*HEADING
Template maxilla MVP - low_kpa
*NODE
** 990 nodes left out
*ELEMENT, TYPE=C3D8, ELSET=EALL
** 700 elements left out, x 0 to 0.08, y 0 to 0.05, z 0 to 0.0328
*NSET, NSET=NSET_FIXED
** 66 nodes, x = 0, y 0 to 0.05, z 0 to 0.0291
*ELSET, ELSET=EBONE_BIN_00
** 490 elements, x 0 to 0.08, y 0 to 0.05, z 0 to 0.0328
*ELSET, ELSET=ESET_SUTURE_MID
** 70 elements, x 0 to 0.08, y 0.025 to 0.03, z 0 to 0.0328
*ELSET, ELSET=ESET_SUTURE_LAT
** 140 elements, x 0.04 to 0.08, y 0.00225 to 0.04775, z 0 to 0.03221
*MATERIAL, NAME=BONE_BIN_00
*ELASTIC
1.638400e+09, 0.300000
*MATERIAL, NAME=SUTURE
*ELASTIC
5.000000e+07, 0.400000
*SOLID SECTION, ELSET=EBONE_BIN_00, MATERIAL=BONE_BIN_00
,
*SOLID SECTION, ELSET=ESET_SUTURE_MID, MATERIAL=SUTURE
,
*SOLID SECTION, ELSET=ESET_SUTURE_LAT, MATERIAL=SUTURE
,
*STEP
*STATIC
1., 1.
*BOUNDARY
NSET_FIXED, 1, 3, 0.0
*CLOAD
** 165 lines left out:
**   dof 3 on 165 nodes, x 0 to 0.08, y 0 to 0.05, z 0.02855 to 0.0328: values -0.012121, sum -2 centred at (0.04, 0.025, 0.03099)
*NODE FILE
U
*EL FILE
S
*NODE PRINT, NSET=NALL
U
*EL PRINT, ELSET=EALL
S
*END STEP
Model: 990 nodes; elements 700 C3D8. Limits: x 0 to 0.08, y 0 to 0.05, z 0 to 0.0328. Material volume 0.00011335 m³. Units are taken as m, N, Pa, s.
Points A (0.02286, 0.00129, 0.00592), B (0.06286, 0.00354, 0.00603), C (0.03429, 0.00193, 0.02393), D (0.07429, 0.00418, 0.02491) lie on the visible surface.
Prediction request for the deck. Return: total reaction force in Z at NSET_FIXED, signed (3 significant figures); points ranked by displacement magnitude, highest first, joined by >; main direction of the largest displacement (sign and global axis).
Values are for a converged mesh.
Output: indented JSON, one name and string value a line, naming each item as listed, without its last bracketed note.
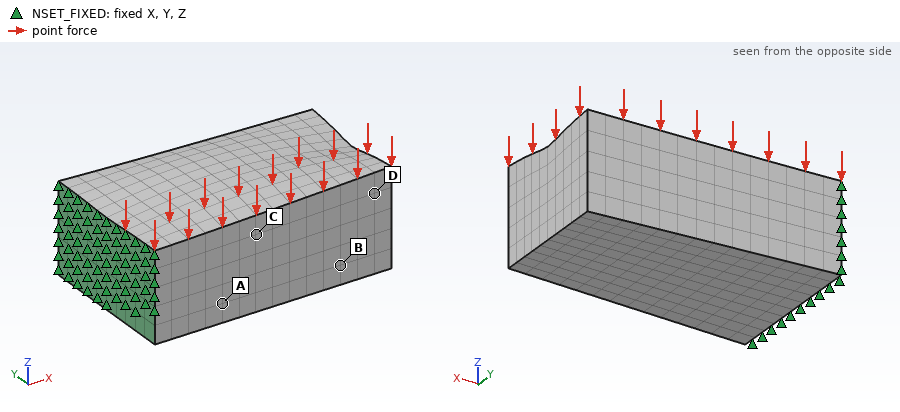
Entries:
{
  "total reaction force in Z at NSET_FIXED, signed": "2.00 N",
  "points ranked by displacement magnitude, highest first, joined by >": "D > B > C > A",
  "main direction of the largest displacement": "-Z"
}
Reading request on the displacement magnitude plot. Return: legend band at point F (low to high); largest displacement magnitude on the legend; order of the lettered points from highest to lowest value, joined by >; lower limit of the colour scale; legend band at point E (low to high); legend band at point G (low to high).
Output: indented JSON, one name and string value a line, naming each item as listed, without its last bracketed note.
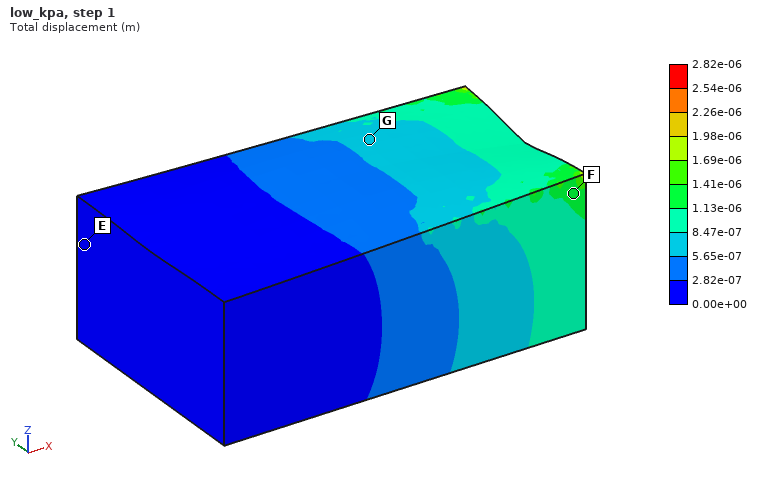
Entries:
{
  "legend band at point F": "1.13e-06 to 1.41e-06 m",
  "largest displacement magnitude on the legend": "2.82e-06 m",
  "order of the lettered points from highest to lowest value, joined by >": "F > G > E",
  "lower limit of the colour scale": "0.00e+00 m",
  "legend band at point E": "0.00e+00 to 2.82e-07 m",
  "legend band at point G": "5.65e-07 to 8.47e-07 m"
}
